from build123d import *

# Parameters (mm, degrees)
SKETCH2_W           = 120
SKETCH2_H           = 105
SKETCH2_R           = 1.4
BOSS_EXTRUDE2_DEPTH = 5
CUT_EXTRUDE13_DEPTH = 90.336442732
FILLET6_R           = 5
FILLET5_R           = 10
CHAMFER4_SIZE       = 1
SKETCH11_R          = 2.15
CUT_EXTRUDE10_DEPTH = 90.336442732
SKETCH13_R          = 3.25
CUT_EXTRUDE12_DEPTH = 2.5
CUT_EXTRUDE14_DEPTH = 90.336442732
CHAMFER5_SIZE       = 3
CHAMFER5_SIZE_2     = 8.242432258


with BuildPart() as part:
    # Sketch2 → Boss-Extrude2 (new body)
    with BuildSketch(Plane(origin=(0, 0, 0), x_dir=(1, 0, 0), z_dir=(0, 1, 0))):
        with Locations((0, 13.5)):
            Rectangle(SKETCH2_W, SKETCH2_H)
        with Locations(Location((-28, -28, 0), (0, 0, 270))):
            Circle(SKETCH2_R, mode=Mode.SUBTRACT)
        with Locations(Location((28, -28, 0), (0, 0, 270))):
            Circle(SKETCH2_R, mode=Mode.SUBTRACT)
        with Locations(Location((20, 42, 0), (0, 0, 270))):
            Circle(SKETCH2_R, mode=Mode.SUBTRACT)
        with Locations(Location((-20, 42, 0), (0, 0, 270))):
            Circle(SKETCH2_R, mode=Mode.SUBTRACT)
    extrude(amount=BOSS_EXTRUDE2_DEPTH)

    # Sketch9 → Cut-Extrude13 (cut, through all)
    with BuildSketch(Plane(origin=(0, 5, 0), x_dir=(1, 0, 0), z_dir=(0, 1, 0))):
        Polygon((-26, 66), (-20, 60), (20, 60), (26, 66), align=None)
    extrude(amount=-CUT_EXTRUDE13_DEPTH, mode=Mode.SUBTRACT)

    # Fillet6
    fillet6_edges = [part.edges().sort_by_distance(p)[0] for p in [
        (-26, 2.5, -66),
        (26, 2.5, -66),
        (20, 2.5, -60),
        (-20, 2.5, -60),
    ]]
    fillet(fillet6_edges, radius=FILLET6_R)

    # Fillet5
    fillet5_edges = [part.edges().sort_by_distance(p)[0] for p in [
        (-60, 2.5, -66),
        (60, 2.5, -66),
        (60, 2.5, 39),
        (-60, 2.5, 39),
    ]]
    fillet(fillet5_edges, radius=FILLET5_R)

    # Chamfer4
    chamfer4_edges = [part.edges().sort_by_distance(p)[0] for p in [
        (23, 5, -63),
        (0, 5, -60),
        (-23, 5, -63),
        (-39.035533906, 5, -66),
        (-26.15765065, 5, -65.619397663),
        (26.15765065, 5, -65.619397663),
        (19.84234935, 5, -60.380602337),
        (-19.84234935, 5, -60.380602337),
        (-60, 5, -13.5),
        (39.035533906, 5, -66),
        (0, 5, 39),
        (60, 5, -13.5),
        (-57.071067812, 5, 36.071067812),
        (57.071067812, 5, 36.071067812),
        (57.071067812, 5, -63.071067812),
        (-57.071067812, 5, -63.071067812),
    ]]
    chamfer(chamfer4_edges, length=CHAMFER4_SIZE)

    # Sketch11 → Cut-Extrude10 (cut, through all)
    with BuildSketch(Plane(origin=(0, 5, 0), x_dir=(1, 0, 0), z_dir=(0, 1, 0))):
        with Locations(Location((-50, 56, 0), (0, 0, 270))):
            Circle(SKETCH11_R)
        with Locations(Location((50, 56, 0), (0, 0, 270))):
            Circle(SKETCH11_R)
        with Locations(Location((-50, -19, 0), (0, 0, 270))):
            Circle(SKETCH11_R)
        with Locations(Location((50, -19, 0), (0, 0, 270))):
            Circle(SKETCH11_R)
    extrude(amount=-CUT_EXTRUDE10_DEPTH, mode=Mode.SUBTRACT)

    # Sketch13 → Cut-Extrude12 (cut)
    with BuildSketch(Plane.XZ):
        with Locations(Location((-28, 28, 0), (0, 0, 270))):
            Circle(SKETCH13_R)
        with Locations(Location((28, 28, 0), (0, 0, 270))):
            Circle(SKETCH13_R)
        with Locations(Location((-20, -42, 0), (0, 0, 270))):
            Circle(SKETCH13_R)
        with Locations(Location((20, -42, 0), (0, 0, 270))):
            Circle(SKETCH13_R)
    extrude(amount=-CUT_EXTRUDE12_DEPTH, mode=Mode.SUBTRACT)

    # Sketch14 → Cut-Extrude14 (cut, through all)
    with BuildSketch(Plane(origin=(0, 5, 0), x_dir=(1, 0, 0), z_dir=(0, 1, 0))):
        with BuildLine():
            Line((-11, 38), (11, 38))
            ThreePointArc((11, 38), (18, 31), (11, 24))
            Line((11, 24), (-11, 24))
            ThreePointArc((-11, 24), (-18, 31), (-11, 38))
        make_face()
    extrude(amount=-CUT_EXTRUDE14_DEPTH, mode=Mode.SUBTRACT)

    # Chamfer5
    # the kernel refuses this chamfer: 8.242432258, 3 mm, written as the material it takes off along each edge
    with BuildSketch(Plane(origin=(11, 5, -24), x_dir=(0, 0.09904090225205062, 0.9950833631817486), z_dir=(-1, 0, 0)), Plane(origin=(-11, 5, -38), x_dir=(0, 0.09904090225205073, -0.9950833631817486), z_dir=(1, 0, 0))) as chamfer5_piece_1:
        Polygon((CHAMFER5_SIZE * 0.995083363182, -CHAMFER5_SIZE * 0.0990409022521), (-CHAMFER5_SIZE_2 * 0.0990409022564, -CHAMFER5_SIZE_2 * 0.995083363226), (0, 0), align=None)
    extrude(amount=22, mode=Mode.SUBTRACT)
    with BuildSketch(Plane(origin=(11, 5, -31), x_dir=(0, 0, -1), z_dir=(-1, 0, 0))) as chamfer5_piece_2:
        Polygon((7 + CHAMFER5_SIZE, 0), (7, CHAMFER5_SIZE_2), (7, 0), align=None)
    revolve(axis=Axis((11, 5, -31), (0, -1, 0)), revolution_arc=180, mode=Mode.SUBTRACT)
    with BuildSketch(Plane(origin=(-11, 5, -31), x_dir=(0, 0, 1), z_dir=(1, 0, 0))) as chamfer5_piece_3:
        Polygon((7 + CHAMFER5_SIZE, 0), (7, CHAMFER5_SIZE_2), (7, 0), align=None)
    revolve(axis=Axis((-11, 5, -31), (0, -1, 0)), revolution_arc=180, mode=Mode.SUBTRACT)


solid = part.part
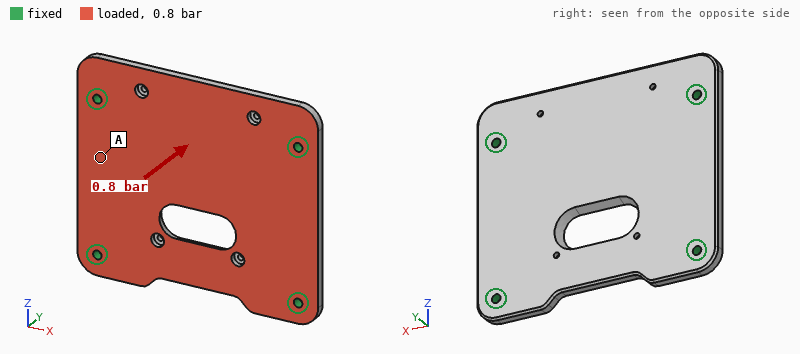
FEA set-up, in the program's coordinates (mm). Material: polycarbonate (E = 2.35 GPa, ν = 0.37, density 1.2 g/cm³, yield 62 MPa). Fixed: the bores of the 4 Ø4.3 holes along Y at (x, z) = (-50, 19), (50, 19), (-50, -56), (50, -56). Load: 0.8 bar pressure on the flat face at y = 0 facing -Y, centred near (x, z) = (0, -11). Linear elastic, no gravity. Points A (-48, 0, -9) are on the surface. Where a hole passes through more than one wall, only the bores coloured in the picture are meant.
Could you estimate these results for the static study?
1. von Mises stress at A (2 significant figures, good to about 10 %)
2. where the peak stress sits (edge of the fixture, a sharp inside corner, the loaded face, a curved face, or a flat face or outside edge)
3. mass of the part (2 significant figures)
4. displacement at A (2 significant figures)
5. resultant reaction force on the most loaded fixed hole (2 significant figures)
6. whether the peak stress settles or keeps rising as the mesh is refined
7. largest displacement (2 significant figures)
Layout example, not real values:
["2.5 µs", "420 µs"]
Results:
["5.1 MPa", "edge of the fixture", "68 g", "0.41 mm", "270 N", "keeps rising", "1.7 mm"]
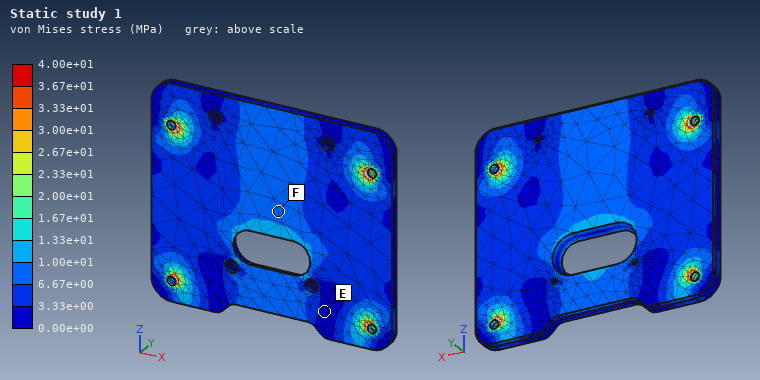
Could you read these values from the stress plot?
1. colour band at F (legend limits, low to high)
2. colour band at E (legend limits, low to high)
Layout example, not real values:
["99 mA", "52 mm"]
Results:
["6.67e+00 to 1.00e+01 MPa", "0.00e+00 to 3.33e+00 MPa"]
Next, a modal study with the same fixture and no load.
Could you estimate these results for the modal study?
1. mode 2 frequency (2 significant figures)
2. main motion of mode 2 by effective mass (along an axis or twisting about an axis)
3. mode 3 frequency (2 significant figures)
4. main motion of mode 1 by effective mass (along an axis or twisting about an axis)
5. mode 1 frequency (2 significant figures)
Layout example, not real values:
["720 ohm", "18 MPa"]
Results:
["780 Hz", "twisting about X", "1100 Hz", "along Y", "580 Hz"]
